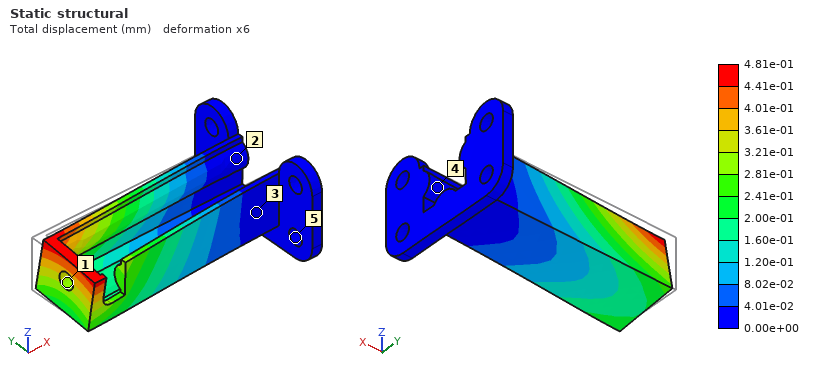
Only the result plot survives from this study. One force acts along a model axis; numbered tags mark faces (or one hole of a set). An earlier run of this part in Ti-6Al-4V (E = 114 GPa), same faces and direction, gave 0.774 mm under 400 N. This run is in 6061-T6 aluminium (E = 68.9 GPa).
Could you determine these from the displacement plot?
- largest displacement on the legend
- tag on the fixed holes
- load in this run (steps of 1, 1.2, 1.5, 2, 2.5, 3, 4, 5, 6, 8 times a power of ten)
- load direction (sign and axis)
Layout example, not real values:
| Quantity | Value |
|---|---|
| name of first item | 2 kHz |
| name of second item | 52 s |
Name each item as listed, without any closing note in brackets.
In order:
| Quantity | Value |
|---|---|
| largest displacement on the legend | 4.81e-01 mm |
| tag on the fixed holes | 5 |
| load in this run | 150 N |
| load direction | -Y |
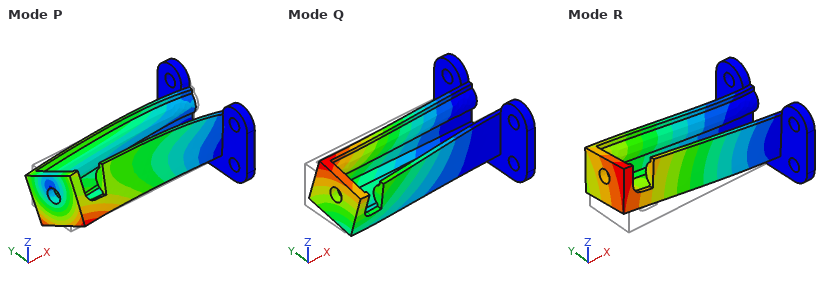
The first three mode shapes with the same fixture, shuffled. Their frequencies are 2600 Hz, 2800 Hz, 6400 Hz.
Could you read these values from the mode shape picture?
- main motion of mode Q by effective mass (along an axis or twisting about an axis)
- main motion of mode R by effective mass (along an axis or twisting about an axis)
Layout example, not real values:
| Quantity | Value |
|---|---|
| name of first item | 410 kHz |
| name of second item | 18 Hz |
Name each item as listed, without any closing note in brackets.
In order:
| Quantity | Value |
|---|---|
| main motion of mode Q by effective mass | along Y |
| main motion of mode R by effective mass | along Z |
